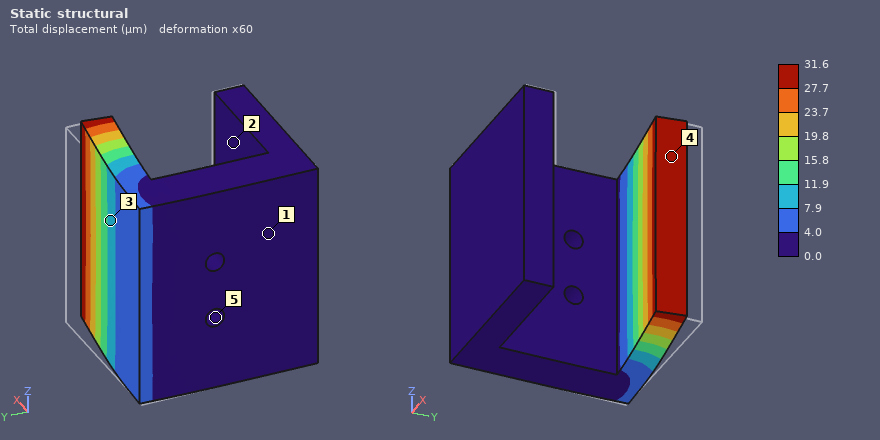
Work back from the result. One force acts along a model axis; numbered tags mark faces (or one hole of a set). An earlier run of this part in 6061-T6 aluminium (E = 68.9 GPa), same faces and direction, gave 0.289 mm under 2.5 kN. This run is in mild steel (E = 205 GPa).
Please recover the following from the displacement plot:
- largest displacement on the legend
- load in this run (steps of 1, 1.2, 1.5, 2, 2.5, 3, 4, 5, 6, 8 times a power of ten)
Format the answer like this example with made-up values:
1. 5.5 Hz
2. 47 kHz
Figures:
1. 31.6 µm
2. 800 N
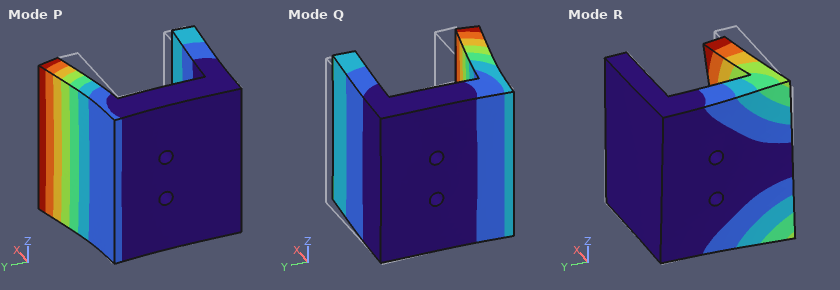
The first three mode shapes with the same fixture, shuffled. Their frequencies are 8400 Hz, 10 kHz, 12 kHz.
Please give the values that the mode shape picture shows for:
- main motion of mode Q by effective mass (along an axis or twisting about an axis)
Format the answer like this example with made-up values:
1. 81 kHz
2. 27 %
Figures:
1. along Y
